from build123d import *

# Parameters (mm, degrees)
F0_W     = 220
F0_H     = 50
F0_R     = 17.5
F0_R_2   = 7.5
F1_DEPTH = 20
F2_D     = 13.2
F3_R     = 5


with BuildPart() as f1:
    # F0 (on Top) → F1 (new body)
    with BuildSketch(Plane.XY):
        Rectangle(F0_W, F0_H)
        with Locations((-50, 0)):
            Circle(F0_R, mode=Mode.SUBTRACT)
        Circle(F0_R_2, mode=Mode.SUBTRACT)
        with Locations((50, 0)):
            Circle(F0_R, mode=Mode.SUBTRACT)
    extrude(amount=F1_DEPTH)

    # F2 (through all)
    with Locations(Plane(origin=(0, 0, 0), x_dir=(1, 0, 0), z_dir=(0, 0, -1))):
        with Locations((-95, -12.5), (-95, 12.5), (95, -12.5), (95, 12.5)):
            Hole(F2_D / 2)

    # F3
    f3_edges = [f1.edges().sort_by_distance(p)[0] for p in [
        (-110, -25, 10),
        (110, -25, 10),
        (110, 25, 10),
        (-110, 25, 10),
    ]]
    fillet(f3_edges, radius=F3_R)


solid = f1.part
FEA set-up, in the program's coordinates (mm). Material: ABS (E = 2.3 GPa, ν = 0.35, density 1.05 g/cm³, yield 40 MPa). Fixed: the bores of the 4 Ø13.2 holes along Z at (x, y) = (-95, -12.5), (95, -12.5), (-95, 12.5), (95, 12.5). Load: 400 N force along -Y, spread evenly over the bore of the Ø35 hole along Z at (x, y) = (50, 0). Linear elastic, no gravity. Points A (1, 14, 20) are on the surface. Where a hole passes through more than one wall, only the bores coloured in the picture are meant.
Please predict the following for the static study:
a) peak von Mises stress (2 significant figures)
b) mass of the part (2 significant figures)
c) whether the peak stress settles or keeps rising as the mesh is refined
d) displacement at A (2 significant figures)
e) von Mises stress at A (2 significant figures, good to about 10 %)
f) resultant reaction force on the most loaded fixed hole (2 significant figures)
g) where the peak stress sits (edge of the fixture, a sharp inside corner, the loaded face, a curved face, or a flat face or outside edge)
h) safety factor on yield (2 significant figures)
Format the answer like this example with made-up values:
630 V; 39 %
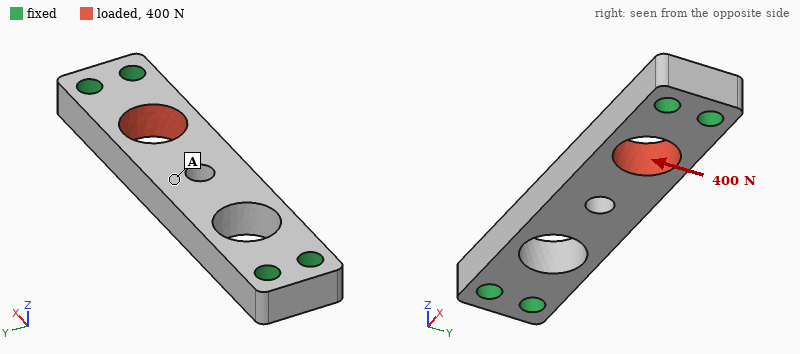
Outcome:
2.7 MPa; 170 g; settles; 77 µm; 0.35 MPa; 260 N; the loaded face; 15
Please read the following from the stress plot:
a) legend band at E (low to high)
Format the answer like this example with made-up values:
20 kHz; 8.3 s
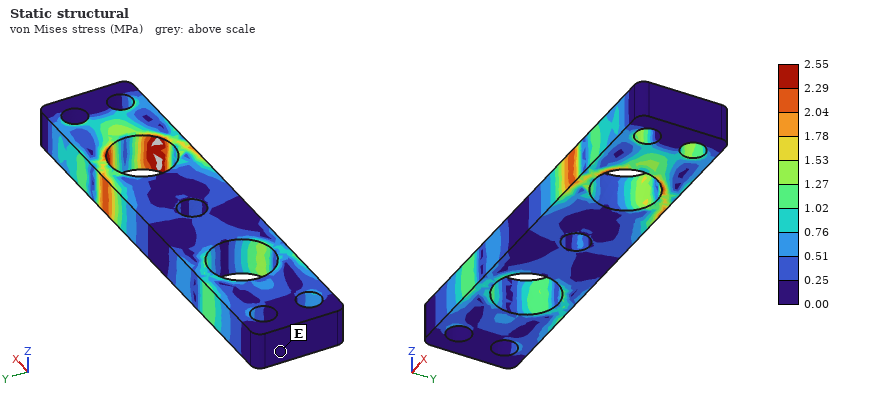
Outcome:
0.00 to 0.25 MPa
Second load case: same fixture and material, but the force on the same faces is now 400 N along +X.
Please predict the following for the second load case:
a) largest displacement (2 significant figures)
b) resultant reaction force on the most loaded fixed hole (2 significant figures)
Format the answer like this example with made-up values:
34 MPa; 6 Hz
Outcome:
11 µm; 150 N
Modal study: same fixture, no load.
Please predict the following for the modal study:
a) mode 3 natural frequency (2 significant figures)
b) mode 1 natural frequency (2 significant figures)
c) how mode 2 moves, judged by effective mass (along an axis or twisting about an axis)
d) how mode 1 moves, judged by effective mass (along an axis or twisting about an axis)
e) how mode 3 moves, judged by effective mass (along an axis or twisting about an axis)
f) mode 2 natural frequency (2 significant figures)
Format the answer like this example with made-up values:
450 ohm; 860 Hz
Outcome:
1300 Hz; 820 Hz; along Y; along Z; twisting about X; 950 Hz
